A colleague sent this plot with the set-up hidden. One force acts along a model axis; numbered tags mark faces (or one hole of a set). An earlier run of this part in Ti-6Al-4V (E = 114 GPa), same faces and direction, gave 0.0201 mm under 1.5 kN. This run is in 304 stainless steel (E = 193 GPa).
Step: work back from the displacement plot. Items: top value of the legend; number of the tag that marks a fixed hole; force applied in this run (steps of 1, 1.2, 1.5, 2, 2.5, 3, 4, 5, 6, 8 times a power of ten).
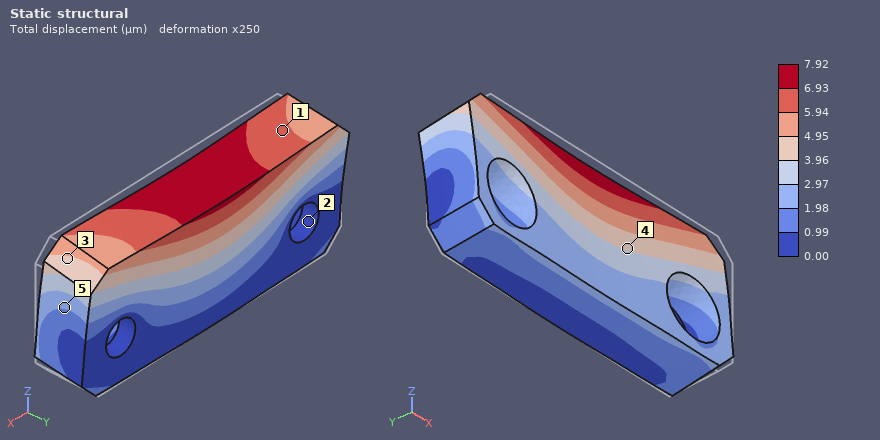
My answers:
7.92 µm
2
1 kN
